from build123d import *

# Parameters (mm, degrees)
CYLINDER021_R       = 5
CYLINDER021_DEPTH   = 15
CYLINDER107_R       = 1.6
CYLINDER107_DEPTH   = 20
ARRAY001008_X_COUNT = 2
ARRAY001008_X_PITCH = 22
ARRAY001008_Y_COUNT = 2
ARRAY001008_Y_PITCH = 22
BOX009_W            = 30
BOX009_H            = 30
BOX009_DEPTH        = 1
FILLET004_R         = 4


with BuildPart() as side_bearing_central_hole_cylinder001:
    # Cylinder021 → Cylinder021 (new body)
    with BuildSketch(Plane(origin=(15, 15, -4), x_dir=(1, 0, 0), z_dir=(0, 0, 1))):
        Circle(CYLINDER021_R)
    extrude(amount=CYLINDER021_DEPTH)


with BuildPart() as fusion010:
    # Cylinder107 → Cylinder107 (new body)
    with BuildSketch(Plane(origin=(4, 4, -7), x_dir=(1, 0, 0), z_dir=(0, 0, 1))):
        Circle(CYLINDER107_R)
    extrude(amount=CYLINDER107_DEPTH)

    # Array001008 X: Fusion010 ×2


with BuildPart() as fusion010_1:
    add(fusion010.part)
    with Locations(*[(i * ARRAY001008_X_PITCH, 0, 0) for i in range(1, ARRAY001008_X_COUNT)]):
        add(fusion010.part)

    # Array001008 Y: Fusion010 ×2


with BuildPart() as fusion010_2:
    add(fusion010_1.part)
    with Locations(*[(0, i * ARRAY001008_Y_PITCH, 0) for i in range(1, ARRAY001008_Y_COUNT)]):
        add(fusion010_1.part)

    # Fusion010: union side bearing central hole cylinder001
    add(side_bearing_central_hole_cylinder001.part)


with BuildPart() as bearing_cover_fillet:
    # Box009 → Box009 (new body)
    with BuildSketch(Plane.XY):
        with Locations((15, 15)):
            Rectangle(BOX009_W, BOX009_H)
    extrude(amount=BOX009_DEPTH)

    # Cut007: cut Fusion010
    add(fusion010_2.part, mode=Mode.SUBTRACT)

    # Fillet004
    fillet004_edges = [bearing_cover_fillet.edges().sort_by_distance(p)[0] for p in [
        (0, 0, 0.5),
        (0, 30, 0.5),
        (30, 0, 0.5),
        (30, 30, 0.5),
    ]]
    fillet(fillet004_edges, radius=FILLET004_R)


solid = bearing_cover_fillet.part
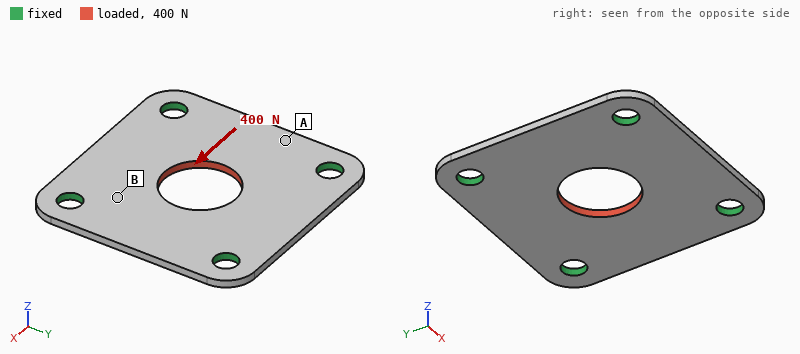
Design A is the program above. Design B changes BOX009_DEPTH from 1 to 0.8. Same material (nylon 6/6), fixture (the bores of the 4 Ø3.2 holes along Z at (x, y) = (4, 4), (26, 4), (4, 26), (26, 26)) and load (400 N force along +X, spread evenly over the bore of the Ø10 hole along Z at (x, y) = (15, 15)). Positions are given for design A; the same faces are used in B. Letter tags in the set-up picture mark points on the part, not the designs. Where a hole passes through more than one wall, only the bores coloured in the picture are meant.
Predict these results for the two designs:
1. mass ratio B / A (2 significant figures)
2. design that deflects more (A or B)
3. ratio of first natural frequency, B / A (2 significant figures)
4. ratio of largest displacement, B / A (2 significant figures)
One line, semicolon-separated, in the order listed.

0.80; B; 0.81; 1.2
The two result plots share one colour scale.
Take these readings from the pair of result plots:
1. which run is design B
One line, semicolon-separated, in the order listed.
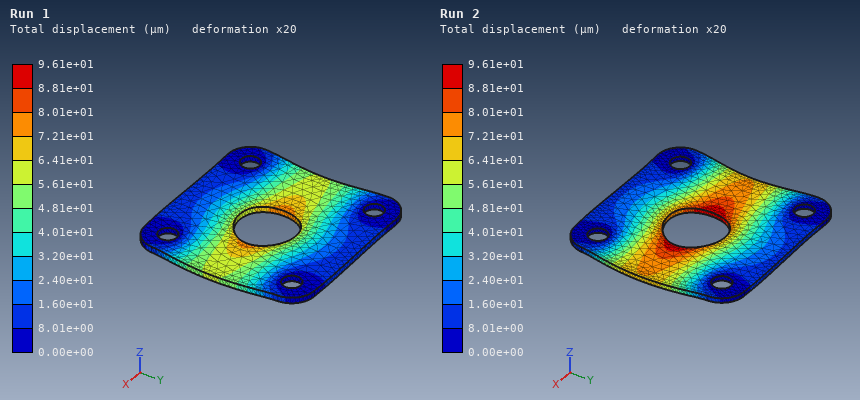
Run 2
